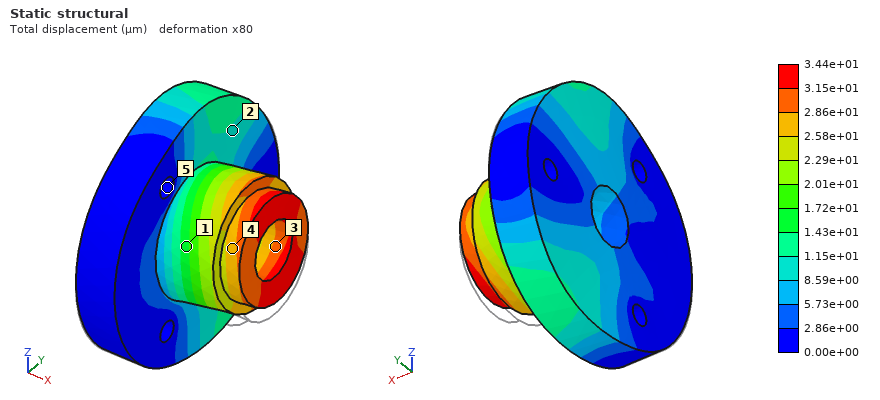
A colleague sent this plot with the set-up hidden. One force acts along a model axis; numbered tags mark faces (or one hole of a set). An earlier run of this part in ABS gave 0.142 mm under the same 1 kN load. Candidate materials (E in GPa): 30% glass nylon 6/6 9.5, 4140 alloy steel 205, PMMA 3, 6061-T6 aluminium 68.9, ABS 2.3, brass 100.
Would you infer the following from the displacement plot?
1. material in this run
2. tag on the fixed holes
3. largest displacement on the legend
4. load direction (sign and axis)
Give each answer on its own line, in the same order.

30% glass nylon 6/6
5
3.44e+01 µm
+Z
